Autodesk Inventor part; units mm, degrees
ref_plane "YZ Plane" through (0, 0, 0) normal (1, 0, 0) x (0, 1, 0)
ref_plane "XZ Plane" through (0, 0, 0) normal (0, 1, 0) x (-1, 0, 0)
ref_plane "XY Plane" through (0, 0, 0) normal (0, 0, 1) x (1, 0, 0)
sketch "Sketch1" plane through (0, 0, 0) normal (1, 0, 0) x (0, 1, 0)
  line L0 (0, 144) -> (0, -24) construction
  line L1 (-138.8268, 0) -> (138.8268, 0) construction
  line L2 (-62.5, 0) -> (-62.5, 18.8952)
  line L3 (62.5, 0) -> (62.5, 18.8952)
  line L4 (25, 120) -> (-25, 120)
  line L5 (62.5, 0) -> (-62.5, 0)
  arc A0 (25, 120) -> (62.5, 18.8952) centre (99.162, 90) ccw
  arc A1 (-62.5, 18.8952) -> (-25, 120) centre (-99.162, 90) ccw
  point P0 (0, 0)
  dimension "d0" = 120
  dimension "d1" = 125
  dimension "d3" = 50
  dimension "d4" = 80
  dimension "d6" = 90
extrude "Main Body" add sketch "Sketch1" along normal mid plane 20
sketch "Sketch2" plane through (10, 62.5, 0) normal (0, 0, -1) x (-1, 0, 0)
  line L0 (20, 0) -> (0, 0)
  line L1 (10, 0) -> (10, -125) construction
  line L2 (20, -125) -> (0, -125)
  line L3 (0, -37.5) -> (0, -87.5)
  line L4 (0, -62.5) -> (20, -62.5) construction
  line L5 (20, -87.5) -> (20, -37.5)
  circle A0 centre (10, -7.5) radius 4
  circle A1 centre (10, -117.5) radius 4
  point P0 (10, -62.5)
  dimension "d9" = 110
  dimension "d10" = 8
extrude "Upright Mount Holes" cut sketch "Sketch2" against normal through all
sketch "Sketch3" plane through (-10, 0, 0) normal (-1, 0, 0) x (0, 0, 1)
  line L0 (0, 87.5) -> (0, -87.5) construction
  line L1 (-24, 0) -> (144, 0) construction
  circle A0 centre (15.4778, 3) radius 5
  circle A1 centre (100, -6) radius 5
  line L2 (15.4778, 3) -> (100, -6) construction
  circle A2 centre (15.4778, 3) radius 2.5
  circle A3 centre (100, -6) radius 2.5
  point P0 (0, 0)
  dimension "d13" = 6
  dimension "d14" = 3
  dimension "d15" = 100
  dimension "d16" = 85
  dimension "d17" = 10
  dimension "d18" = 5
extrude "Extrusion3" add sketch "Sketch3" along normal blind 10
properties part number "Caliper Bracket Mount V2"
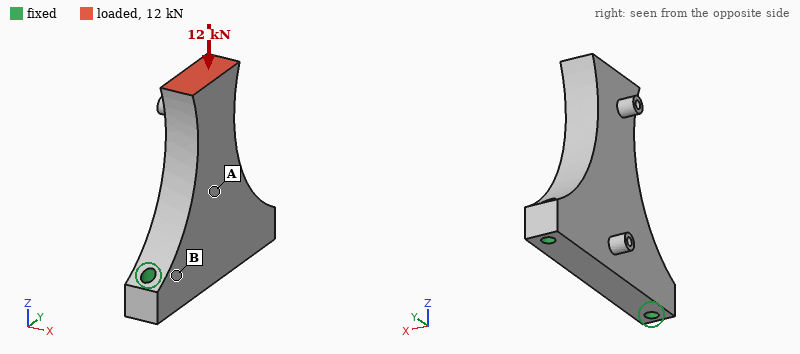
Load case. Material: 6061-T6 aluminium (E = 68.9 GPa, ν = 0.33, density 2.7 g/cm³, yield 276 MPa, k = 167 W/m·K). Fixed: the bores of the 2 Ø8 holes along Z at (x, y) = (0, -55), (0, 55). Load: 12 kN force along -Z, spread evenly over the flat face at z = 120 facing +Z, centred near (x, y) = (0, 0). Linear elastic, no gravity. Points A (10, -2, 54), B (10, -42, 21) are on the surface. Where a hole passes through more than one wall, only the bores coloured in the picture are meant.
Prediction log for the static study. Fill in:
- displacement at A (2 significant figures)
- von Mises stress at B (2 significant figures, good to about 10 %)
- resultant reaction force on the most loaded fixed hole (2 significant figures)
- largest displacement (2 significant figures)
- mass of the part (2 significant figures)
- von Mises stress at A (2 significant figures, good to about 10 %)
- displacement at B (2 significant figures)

19 µm
19 MPa
6.9 kN
36 µm
440 g
8.1 MPa
6.7 µm
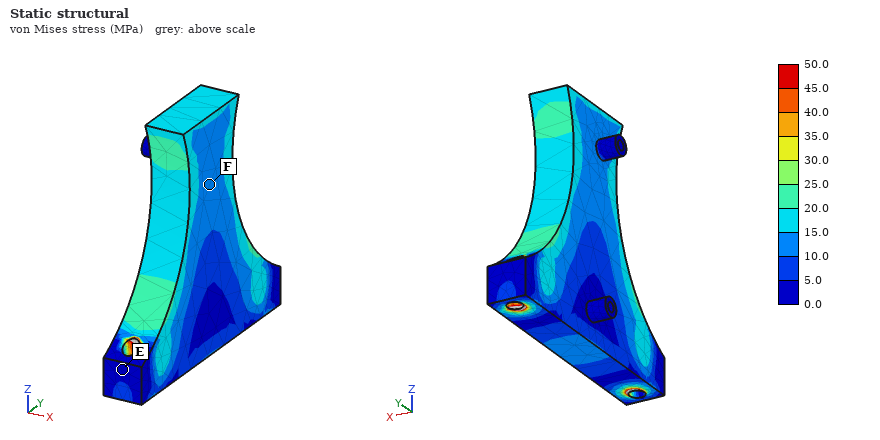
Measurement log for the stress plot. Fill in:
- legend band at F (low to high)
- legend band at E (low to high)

10.0 to 15.0 MPa
0.0 to 5.0 MPa
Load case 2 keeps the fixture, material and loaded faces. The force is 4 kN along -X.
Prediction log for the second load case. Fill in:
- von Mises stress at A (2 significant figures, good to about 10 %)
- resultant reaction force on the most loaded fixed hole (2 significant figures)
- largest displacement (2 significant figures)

78 MPa
2.0 kN
0.97 mm
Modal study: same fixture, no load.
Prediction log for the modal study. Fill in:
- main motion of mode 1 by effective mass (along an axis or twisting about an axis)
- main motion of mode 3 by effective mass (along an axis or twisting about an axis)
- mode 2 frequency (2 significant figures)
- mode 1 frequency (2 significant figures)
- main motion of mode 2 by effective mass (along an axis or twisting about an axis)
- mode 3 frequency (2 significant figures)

along X
along X
4500 Hz
1200 Hz
along Y
5200 Hz
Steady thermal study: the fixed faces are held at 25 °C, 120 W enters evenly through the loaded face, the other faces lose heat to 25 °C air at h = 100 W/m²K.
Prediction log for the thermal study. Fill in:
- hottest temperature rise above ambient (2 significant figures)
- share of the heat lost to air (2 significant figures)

68 K
42 %
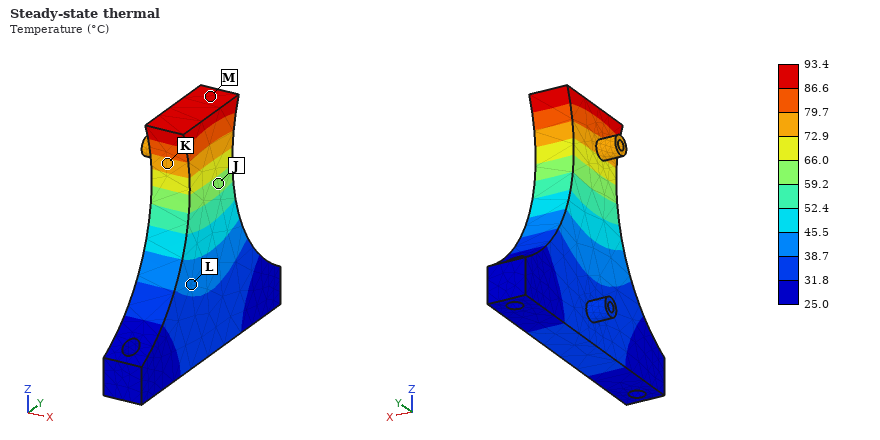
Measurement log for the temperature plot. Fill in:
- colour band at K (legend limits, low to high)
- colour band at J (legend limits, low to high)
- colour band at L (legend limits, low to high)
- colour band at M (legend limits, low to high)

72.9 to 79.7 °C
59.2 to 66.0 °C
38.7 to 45.5 °C
86.6 to 93.4 °C
